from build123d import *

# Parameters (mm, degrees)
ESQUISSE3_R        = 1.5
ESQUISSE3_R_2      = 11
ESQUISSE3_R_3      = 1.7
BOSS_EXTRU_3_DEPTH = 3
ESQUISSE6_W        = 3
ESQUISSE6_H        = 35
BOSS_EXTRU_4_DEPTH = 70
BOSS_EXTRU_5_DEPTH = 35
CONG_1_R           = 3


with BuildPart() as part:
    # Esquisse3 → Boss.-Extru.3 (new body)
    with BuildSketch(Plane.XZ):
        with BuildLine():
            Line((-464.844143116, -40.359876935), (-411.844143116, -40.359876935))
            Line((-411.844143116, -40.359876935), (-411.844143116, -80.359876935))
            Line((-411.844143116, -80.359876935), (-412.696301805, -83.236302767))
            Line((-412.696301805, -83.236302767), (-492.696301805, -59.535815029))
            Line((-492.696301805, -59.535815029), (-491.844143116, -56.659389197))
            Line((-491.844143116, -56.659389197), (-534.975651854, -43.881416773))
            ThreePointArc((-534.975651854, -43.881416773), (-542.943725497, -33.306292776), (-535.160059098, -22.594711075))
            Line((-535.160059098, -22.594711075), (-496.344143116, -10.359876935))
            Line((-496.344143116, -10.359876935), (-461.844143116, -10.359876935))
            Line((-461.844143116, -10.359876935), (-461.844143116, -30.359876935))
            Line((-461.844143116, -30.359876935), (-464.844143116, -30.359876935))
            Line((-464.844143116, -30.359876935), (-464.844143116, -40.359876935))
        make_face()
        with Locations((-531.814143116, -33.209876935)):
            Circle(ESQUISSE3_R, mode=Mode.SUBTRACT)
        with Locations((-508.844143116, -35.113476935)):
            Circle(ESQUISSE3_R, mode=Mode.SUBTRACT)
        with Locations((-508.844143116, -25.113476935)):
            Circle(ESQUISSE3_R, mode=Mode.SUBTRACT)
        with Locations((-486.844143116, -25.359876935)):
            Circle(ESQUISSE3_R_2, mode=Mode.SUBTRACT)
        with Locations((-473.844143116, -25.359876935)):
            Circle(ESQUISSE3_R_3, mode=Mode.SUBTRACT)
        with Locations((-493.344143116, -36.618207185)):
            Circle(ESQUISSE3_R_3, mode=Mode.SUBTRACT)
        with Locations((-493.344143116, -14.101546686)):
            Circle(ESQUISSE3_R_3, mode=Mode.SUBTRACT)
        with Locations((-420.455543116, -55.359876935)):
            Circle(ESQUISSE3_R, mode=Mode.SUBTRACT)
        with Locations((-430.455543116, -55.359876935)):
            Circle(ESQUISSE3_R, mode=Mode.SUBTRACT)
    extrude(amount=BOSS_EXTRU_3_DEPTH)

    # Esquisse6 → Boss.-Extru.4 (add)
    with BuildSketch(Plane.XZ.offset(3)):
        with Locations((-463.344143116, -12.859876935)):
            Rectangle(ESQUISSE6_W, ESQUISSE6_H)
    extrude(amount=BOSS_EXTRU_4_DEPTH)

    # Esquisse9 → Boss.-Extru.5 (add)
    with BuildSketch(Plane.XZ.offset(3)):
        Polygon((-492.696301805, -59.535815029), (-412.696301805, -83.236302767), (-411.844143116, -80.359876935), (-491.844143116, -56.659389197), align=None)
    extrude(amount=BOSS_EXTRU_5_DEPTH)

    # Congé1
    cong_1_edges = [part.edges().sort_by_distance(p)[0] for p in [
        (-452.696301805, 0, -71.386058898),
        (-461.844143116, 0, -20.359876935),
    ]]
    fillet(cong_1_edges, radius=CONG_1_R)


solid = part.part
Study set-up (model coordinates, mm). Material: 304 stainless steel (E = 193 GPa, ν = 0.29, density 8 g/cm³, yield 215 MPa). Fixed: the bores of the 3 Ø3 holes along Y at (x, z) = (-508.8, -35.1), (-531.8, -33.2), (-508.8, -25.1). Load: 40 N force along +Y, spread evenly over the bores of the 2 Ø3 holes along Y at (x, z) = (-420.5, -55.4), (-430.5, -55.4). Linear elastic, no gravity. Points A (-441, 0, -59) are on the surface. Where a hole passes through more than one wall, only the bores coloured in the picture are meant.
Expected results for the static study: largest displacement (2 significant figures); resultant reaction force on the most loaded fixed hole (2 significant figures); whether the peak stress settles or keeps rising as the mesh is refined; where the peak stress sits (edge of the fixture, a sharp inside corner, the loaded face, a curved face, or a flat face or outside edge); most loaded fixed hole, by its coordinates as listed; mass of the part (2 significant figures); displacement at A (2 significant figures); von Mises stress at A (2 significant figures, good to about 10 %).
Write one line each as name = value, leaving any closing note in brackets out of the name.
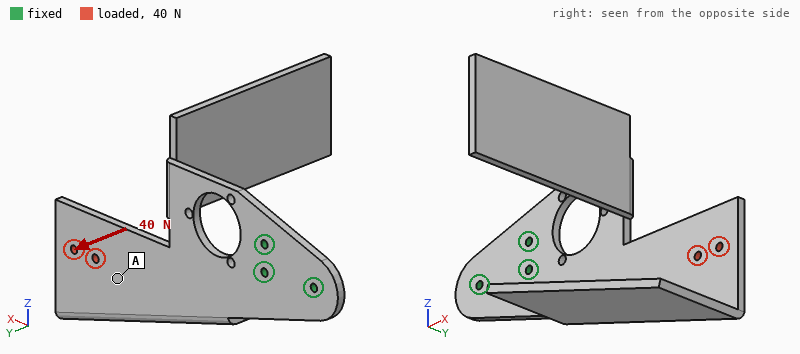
largest displacement = 0.77 mm
resultant reaction force on the most loaded fixed hole = 130 N
whether the peak stress settles or keeps rising as the mesh is refined = keeps rising
where the peak stress sits = a sharp inside corner
most loaded fixed hole, by its coordinates as listed = (-508.8, -35.1)
mass of the part = 240 g
displacement at A = 0.46 mm
von Mises stress at A = 9.5 MPa
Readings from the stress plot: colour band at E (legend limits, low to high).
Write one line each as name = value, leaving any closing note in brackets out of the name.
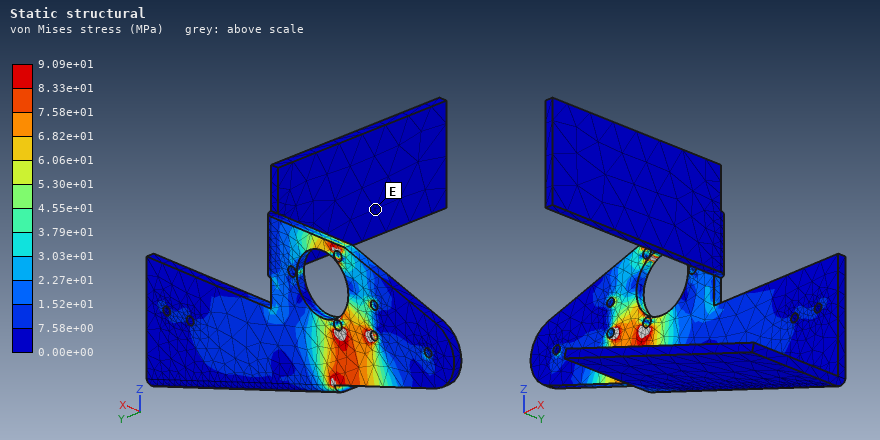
colour band at E = 0.00e+00 to 7.58e+00 MPa
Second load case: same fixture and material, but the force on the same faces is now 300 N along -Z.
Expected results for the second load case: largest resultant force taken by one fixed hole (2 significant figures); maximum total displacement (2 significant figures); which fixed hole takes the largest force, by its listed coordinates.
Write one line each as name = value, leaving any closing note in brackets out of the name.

largest resultant force taken by one fixed hole = 960 N
maximum total displacement = 0.10 mm
which fixed hole takes the largest force, by its listed coordinates = (-508.8, -25.1)
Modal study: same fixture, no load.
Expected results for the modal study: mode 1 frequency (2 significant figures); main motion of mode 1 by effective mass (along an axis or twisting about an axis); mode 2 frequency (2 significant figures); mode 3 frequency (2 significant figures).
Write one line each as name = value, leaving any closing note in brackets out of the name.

mode 1 frequency = 130 Hz
main motion of mode 1 by effective mass = along Y
mode 2 frequency = 200 Hz
mode 3 frequency = 350 Hz
